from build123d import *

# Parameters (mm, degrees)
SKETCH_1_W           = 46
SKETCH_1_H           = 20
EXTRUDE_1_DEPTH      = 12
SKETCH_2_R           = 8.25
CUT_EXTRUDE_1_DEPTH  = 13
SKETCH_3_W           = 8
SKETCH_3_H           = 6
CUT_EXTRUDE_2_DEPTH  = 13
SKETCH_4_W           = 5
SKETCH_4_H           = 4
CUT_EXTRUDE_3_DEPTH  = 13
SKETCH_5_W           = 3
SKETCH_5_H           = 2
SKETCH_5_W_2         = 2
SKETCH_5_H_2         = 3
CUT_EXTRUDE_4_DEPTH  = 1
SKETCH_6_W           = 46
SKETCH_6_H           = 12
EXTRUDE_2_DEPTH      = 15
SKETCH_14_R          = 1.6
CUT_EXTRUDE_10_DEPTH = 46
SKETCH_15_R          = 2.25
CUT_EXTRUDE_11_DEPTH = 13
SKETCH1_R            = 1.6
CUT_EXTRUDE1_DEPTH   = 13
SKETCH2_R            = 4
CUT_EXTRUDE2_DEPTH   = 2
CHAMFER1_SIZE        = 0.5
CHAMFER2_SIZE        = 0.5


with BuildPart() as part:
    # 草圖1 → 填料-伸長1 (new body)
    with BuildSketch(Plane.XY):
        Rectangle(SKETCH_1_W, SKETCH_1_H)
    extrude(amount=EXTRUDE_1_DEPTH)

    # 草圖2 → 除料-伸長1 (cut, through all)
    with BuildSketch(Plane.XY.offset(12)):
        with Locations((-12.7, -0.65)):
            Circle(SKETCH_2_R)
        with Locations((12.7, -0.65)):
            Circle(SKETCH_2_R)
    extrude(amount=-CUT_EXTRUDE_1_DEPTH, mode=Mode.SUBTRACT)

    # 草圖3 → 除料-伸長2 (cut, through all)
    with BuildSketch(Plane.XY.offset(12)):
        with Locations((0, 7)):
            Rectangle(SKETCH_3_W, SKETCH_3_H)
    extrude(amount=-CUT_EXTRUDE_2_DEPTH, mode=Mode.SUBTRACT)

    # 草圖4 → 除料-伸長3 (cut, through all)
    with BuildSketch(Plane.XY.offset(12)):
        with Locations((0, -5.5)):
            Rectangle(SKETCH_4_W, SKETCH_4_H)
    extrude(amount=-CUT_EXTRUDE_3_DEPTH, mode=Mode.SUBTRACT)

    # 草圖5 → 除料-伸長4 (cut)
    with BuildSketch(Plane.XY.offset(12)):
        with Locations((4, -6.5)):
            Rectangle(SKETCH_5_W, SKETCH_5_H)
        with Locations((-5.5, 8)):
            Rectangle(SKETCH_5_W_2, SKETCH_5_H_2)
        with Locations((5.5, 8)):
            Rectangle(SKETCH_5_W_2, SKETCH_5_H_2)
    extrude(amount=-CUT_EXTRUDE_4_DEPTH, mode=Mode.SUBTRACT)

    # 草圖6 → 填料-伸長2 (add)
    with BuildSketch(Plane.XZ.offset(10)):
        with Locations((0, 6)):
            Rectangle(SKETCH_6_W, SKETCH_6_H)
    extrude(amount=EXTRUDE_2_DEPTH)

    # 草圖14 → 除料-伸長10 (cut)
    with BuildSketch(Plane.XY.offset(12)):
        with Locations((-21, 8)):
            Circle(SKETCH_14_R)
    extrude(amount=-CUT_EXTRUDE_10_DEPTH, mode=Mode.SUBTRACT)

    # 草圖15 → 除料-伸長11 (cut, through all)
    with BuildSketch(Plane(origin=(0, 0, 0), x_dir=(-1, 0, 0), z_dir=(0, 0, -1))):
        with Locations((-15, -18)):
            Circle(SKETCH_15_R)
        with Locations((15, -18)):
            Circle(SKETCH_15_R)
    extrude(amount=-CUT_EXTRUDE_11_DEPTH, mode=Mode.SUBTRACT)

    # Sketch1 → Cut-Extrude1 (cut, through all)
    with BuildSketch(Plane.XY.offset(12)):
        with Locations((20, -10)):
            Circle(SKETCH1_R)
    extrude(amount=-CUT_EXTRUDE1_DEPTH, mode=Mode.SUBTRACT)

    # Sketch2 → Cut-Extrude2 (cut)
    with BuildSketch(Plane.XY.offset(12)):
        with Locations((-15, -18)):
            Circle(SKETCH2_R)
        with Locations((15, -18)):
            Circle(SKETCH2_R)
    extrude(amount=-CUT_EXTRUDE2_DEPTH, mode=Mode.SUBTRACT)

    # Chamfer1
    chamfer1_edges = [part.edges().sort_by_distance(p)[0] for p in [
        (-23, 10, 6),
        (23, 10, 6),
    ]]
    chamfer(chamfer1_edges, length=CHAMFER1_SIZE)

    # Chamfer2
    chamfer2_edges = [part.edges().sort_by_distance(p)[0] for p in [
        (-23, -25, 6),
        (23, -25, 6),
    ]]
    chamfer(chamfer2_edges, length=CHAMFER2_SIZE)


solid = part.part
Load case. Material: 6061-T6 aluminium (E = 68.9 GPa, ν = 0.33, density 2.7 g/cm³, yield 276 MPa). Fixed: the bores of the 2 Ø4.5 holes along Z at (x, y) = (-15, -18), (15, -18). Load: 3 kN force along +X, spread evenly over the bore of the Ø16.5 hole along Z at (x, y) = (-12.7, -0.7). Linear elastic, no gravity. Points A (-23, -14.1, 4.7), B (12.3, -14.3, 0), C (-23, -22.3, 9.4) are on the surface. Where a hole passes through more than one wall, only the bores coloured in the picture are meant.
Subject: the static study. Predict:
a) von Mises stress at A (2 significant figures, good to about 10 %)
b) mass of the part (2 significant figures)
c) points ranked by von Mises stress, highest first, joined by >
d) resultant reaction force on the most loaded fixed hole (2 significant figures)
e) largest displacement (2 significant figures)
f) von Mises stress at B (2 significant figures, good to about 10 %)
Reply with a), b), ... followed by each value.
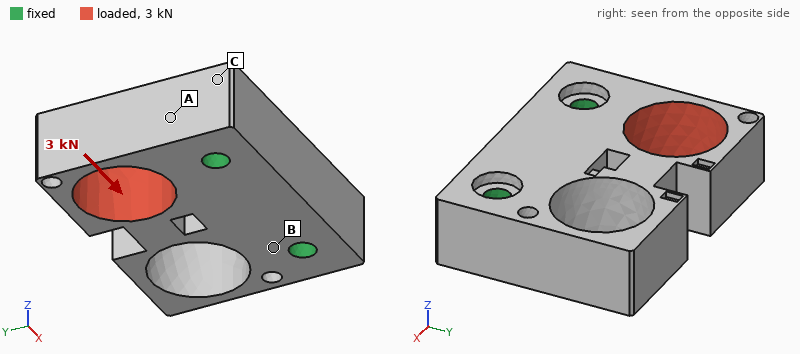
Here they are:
a) 36 MPa
b) 34 g
c) A > B > C
d) 2.2 kN
e) 58 µm
f) 25 MPa
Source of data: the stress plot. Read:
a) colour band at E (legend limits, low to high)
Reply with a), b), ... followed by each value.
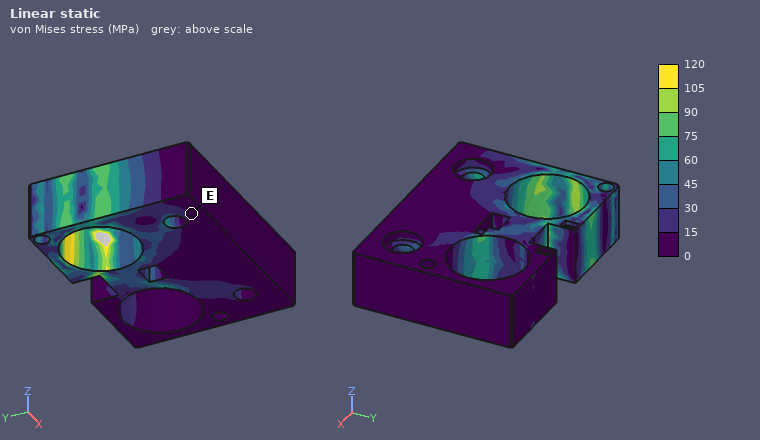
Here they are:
a) 0 to 15 MPa
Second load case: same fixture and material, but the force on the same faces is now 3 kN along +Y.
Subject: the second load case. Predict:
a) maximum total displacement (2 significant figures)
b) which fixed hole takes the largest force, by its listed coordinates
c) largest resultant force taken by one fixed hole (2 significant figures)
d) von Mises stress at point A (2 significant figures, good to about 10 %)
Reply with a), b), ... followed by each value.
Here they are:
a) 30 µm
b) (-15, -18)
c) 2.6 kN
d) 27 MPa
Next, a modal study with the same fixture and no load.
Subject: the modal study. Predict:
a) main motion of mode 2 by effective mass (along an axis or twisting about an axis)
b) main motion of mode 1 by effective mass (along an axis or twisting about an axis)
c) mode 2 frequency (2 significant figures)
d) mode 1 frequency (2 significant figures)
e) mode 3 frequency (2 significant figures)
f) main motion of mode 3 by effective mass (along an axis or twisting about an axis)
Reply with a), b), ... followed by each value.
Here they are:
a) twisting about Y
b) along Z
c) 13 kHz
d) 9300 Hz
e) 14 kHz
f) along X
